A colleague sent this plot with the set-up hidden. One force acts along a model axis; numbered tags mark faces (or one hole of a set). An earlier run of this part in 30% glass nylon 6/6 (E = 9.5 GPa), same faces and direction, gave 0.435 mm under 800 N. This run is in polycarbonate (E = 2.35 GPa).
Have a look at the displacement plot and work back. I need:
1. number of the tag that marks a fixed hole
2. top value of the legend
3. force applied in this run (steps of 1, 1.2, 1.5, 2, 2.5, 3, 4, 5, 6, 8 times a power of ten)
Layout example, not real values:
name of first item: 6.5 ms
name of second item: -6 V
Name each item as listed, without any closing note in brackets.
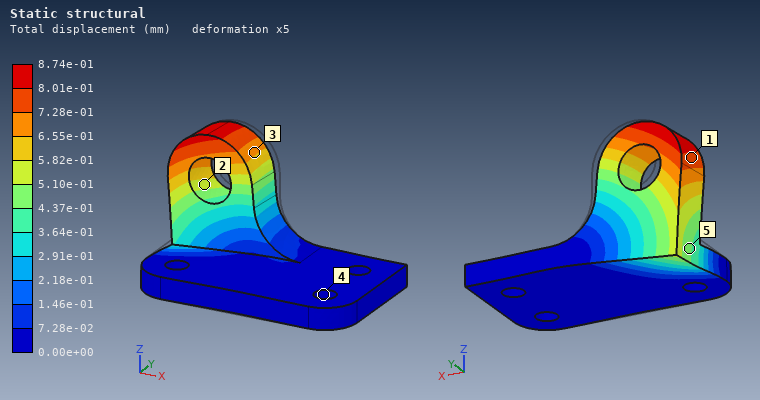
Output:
number of the tag that marks a fixed hole: 4
top value of the legend: 8.74e-01 mm
force applied in this run: 400 N
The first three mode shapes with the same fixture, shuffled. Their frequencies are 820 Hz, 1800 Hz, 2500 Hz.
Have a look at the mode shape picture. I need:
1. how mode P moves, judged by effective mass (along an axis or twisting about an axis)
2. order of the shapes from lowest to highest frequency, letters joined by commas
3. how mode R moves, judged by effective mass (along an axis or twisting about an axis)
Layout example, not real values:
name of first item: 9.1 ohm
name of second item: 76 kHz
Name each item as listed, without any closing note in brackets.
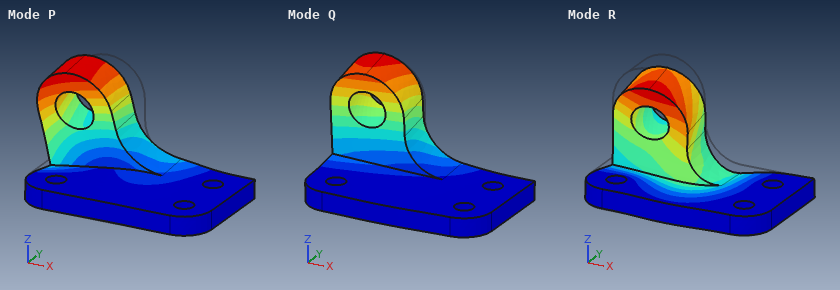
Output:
how mode P moves, judged by effective mass: along X
order of the shapes from lowest to highest frequency, letters joined by commas: Q, P, R
how mode R moves, judged by effective mass: along Z
